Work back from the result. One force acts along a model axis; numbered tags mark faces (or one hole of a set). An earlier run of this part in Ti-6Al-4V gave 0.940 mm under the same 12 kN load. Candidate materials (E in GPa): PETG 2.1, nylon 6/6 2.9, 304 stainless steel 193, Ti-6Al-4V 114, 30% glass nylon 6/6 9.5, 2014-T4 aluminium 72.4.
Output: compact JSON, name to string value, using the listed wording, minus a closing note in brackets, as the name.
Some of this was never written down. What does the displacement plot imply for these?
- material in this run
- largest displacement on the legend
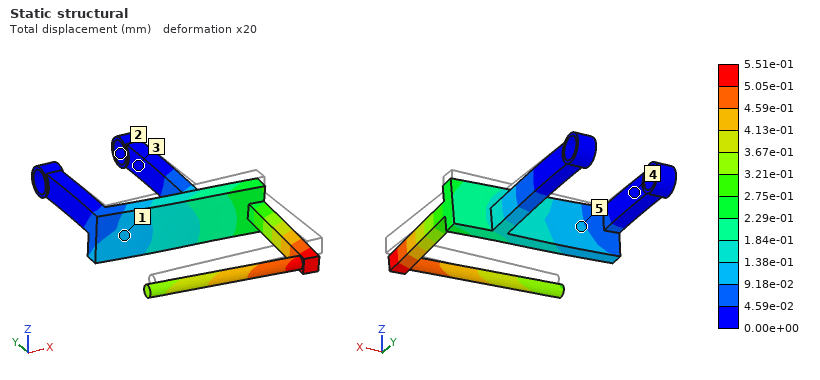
{"material in this run": "304 stainless steel", "largest displacement on the legend": "5.51e-01 mm"}
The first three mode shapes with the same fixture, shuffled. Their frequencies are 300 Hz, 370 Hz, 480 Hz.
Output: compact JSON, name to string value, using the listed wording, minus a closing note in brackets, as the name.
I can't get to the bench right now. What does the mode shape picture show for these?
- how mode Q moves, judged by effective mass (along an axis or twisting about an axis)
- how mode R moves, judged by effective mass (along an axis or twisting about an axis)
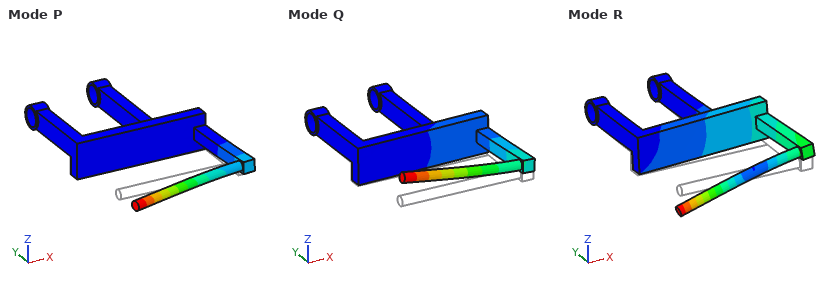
{"how mode Q moves, judged by effective mass": "along Z", "how mode R moves, judged by effective mass": "along Z"}
